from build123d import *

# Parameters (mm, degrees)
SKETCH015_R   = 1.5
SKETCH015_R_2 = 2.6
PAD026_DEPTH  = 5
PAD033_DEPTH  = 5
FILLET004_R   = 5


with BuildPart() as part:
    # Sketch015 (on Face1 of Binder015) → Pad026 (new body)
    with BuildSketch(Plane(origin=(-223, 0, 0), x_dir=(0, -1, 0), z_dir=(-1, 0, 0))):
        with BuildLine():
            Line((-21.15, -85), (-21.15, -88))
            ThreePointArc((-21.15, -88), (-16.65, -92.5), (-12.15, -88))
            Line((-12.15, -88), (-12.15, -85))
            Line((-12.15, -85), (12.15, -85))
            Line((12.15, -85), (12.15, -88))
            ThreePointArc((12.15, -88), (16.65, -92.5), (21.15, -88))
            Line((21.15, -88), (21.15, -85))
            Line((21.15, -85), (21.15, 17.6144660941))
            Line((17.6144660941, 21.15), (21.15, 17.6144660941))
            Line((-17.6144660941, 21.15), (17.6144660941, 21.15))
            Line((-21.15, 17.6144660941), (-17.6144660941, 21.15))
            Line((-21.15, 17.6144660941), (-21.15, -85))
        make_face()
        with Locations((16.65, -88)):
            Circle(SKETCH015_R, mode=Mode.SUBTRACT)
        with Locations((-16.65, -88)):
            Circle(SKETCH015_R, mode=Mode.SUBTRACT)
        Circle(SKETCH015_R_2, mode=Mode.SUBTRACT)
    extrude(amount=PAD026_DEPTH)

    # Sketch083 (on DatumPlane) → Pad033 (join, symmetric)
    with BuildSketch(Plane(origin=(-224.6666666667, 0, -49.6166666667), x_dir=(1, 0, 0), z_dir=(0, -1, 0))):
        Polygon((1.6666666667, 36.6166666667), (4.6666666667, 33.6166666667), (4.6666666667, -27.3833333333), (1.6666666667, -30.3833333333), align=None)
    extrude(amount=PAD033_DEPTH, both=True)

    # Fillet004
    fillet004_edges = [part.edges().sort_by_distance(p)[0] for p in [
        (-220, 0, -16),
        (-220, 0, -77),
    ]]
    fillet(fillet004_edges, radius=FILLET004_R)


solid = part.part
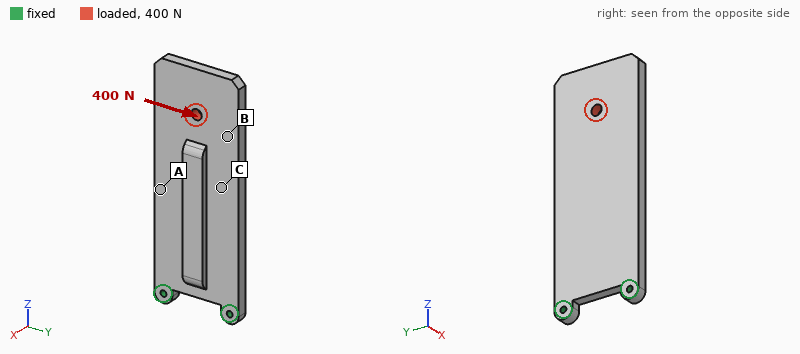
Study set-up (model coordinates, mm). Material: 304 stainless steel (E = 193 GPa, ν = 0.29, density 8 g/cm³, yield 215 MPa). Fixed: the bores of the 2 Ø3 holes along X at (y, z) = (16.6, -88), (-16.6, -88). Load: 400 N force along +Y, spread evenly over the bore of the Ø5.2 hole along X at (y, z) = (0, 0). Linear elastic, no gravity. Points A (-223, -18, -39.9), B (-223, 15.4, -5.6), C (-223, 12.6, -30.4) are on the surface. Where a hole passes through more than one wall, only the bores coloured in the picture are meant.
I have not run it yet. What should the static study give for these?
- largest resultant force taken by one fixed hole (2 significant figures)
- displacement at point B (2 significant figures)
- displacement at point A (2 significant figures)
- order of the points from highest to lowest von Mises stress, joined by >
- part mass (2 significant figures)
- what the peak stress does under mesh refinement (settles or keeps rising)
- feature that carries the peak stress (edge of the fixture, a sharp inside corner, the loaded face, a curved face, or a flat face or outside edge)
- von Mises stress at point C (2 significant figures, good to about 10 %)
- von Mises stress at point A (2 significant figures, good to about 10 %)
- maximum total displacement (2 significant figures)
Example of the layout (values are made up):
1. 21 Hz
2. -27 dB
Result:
1. 1.0 kN
2. 17 µm
3. 8.4 µm
4. A > C > B
5. 200 g
6. keeps rising
7. edge of the fixture
8. 5.3 MPa
9. 9.0 MPa
10. 25 µm
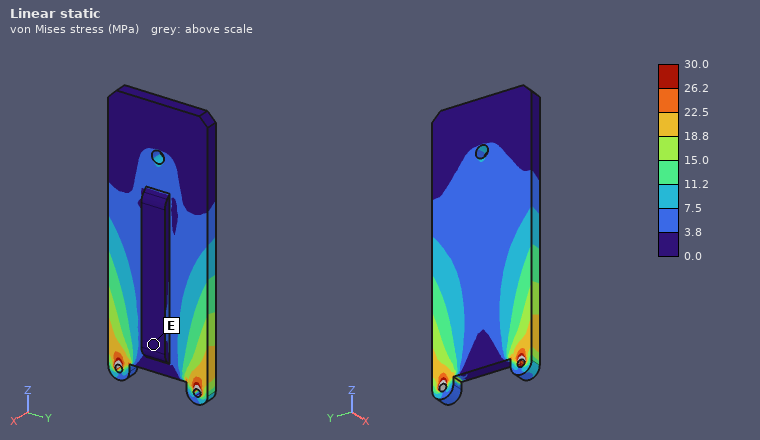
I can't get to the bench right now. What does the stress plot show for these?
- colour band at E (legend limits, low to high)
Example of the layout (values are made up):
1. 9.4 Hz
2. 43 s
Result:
1. 0.0 to 3.8 MPa
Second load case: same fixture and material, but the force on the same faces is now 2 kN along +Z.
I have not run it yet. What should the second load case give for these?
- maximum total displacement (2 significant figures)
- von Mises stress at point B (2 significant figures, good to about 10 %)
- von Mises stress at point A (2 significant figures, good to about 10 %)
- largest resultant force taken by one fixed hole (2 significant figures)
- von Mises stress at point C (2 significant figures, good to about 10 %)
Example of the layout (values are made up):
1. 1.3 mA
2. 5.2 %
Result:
1. 20 µm
2. 5.4 MPa
3. 6.0 MPa
4. 1.0 kN
5. 6.1 MPa
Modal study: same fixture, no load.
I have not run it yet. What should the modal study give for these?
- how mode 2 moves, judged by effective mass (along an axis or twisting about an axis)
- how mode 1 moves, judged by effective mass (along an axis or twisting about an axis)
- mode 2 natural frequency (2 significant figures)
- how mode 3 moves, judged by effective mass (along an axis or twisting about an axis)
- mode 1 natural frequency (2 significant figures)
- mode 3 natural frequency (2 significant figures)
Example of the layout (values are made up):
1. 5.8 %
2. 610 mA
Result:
1. twisting about Z
2. along X
3. 2000 Hz
4. along X
5. 320 Hz
6. 2200 Hz
